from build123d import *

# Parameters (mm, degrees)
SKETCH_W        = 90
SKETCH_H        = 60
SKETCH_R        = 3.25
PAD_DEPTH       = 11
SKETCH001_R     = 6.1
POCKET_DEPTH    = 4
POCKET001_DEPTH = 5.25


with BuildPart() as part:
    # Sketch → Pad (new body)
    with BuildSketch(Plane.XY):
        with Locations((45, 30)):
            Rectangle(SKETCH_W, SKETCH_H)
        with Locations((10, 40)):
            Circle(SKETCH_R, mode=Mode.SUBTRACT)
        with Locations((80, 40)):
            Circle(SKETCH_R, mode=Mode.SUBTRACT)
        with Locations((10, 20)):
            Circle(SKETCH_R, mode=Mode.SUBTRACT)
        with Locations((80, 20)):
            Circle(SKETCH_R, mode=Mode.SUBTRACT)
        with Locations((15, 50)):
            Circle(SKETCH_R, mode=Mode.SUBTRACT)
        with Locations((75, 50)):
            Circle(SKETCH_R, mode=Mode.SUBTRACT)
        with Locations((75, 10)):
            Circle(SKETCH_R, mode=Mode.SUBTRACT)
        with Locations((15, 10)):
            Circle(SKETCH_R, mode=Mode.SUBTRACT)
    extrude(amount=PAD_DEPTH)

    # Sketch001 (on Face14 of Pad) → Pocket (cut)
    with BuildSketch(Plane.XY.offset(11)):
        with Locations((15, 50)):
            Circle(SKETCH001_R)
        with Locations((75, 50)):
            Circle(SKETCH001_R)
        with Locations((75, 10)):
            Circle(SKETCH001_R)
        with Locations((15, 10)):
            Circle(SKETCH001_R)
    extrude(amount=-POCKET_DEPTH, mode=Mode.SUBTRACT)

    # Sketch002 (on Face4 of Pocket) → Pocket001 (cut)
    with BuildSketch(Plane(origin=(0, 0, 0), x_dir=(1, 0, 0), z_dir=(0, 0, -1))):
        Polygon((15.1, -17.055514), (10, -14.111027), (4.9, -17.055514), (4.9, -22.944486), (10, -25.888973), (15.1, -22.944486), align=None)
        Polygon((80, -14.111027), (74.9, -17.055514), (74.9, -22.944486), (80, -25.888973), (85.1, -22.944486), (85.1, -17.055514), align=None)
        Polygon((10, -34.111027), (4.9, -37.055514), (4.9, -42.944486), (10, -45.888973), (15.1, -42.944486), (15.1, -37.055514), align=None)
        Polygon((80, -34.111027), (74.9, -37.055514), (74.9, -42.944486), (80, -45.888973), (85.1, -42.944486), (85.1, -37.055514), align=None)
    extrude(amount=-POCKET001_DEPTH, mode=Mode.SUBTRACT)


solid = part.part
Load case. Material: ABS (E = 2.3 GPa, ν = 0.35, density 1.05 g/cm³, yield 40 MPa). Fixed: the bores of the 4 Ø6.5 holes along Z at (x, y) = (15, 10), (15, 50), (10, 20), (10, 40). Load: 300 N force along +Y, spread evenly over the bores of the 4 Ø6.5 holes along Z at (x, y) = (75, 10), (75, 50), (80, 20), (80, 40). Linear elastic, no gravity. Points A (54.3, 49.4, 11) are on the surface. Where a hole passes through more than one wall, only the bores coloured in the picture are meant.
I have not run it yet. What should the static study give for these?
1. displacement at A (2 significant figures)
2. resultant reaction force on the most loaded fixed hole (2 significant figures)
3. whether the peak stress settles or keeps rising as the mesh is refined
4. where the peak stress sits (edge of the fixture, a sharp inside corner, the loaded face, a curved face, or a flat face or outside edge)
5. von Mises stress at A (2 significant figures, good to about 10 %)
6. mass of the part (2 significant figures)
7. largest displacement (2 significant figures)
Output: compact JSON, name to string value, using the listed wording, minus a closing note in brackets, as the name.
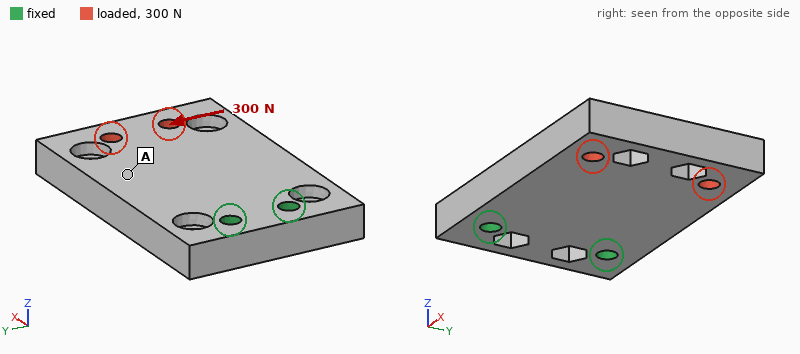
{"displacement at A": "0.065 mm", "resultant reaction force on the most loaded fixed hole": "410 N", "whether the peak stress settles or keeps rising as the mesh is refined": "keeps rising", "where the peak stress sits": "edge of the fixture", "von Mises stress at A": "0.83 MPa", "mass of the part": "57 g", "largest displacement": "0.15 mm"}
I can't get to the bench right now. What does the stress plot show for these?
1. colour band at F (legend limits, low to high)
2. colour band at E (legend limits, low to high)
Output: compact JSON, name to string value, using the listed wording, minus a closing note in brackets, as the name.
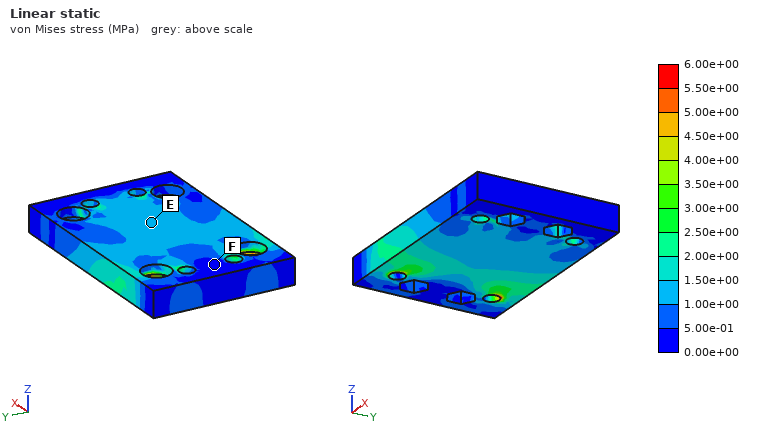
{"colour band at F": "0.00e+00 to 5.00e-01 MPa", "colour band at E": "1.00e+00 to 1.50e+00 MPa"}
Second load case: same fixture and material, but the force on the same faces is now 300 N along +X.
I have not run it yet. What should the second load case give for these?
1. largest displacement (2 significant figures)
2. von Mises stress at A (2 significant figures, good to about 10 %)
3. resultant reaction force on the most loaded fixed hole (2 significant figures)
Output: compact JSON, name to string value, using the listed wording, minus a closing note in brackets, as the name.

{"largest displacement": "29 µm", "von Mises stress at A": "0.44 MPa", "resultant reaction force on the most loaded fixed hole": "92 N"}
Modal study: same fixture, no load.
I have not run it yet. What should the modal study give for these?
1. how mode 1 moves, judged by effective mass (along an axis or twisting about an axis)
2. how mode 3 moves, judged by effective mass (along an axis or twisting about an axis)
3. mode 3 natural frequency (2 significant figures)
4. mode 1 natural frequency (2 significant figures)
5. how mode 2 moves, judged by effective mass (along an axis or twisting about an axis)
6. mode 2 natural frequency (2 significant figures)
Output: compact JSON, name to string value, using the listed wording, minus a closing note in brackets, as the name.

{"how mode 1 moves, judged by effective mass": "along Z", "how mode 3 moves, judged by effective mass": "along Y", "mode 3 natural frequency": "1700 Hz", "mode 1 natural frequency": "440 Hz", "how mode 2 moves, judged by effective mass": "twisting about X", "mode 2 natural frequency": "1200 Hz"}
